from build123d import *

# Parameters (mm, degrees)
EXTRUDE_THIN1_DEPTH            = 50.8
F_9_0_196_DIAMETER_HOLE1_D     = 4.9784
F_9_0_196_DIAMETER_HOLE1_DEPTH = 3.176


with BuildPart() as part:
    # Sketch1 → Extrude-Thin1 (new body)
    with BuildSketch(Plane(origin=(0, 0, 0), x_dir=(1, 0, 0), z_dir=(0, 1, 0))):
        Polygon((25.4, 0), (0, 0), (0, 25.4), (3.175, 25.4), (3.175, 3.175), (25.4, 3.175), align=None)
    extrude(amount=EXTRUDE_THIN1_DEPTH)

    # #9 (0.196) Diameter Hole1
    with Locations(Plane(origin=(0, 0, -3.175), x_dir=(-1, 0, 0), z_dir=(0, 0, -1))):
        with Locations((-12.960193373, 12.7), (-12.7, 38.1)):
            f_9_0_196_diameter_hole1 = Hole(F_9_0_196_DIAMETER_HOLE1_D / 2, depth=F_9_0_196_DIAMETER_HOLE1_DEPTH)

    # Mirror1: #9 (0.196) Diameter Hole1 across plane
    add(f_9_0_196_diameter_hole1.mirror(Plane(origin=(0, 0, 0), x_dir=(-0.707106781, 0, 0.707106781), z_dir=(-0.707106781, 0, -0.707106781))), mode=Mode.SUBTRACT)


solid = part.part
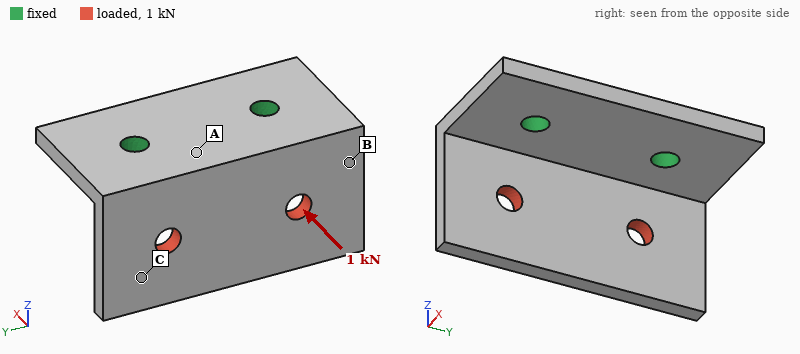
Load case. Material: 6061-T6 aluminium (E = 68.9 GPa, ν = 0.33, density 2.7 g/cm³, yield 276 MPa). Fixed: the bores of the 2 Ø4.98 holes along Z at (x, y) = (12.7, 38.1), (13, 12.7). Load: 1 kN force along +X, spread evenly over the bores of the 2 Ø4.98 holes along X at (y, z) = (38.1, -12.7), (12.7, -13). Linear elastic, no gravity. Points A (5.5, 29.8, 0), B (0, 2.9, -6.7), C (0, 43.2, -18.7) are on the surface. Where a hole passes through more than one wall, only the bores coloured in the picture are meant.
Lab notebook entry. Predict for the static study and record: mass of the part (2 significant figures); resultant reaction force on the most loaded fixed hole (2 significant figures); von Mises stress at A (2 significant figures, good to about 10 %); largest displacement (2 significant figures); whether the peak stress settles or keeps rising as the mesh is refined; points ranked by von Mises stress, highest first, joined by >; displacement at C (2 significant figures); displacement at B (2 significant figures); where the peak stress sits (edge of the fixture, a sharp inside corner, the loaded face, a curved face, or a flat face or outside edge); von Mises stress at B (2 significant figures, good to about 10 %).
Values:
20 g
500 N
110 MPa
0.41 mm
keeps rising
A > B > C
0.29 mm
0.12 mm
edge of the fixture
69 MPa
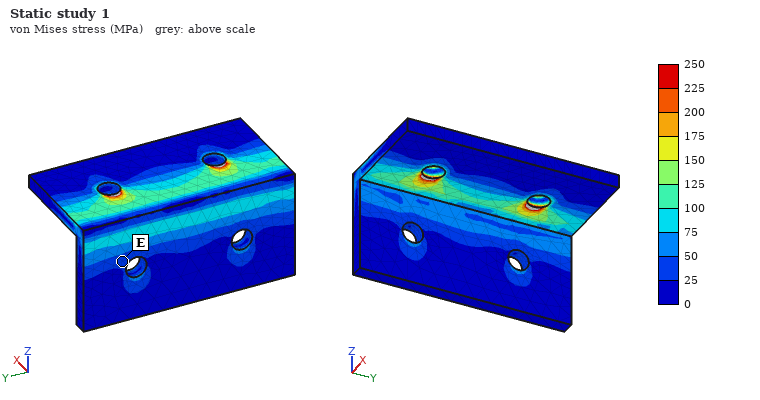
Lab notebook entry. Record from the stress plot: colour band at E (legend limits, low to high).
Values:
25 to 50 MPa
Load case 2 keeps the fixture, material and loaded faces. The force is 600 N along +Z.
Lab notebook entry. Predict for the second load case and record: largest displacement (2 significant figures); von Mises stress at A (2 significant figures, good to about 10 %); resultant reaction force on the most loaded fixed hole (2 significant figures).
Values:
96 µm
24 MPa
300 N
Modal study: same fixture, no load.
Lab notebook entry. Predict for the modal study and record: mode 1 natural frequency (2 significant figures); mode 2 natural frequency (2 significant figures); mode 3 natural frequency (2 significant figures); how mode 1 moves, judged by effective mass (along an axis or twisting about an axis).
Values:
2700 Hz
4600 Hz
7500 Hz
along X
